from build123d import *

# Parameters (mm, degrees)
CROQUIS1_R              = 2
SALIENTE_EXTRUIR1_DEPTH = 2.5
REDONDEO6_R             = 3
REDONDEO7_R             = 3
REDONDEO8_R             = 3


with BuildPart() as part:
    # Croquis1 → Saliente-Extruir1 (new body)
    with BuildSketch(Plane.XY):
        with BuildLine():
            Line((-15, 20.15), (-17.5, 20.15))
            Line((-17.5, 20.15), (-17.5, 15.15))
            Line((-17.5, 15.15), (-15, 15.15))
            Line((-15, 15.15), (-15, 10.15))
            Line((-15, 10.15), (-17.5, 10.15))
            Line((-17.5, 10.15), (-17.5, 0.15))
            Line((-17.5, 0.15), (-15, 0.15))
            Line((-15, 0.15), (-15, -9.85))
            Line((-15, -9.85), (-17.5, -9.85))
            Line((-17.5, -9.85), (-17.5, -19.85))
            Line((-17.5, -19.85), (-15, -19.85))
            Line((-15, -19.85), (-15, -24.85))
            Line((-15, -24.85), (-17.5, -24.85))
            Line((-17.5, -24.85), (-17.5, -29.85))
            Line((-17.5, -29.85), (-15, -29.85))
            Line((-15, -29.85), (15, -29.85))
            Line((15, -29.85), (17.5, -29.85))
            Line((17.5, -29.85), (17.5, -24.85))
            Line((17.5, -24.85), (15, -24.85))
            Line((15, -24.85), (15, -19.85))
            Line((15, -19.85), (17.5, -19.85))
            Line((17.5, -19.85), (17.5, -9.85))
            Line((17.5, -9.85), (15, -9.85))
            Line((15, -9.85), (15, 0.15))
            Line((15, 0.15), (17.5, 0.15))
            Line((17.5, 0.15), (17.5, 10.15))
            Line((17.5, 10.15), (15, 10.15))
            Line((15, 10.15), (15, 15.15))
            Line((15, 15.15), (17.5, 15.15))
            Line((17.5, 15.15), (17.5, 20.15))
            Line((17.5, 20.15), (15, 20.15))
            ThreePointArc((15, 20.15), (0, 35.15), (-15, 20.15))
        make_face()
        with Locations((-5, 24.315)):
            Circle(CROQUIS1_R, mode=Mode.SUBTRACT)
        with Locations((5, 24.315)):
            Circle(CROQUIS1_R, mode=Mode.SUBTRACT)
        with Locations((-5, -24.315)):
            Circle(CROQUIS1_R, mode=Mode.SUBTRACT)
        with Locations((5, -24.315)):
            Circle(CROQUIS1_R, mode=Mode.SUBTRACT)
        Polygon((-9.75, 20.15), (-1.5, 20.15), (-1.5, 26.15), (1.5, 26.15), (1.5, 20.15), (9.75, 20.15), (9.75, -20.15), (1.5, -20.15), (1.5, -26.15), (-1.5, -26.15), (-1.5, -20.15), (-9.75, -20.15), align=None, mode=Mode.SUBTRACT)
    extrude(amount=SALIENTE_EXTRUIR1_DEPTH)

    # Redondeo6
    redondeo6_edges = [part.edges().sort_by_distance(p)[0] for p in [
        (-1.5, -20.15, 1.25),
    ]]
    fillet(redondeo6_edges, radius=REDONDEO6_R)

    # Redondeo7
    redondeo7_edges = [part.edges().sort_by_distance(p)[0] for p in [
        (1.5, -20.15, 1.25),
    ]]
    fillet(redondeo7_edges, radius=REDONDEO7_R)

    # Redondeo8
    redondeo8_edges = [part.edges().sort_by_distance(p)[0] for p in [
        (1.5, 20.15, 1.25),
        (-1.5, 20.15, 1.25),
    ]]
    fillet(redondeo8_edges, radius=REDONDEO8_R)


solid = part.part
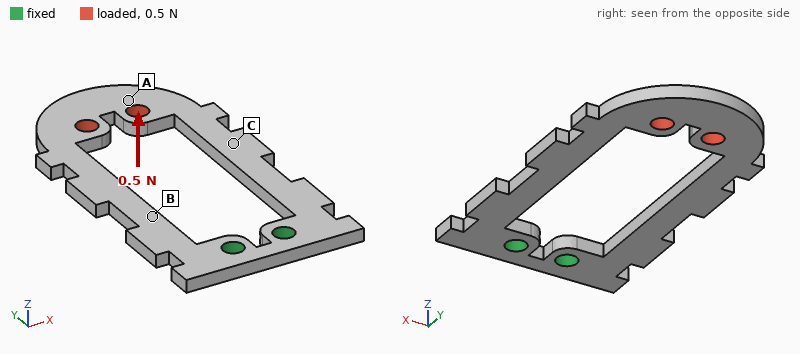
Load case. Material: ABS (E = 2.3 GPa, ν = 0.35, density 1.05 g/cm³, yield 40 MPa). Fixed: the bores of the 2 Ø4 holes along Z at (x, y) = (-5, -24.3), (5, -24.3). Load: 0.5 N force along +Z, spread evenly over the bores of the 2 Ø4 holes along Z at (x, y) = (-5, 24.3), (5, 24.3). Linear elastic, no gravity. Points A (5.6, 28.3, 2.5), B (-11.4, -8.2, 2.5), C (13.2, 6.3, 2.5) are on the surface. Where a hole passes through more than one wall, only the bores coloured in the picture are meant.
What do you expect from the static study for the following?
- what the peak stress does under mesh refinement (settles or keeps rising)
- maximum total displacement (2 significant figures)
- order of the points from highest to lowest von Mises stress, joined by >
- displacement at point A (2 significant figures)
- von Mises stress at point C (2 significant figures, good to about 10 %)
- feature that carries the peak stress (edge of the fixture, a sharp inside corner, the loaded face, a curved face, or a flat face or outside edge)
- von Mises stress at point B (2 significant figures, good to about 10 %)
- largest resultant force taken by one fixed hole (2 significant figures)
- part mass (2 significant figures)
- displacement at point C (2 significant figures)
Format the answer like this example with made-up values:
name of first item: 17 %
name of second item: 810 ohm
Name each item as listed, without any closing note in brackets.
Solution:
what the peak stress does under mesh refinement: keeps rising
maximum total displacement: 0.75 mm
order of the points from highest to lowest von Mises stress, joined by >: B > C > A
displacement at point A: 0.63 mm
von Mises stress at point C: 0.60 MPa
feature that carries the peak stress: a sharp inside corner
von Mises stress at point B: 1.4 MPa
largest resultant force taken by one fixed hole: 0.25 N
part mass: 2.9 g
displacement at point C: 0.27 mm
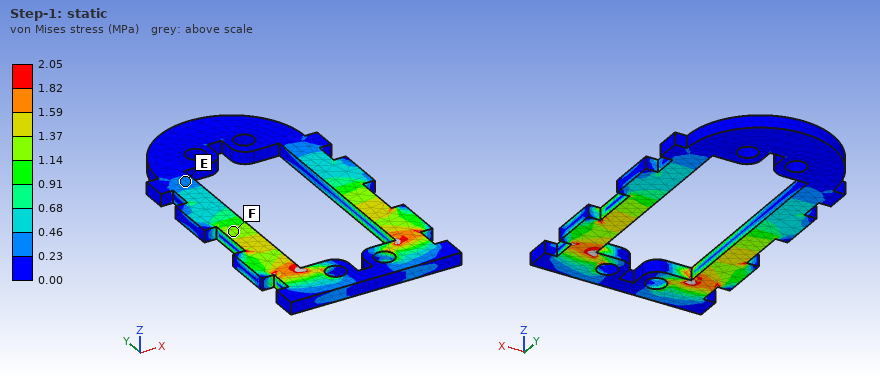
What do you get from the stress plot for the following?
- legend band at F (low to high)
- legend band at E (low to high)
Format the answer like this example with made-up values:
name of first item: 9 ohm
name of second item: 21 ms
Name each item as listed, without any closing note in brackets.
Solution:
legend band at F: 1.14 to 1.37 MPa
legend band at E: 0.23 to 0.46 MPa
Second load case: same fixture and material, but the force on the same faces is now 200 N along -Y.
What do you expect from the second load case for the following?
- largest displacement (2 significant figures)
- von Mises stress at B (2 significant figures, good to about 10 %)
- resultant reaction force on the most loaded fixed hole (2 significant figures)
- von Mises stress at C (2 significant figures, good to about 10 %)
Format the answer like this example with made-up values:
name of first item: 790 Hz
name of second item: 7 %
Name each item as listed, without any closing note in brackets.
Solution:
largest displacement: 0.44 mm
von Mises stress at B: 8.3 MPa
resultant reaction force on the most loaded fixed hole: 110 N
von Mises stress at C: 5.7 MPa
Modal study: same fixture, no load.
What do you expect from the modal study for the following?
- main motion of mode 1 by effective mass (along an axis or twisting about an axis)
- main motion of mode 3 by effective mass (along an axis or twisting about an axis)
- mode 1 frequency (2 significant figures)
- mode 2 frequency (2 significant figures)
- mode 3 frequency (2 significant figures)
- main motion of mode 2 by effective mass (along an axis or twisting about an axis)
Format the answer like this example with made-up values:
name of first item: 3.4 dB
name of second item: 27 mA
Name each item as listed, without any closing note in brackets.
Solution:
main motion of mode 1 by effective mass: along Z
main motion of mode 3 by effective mass: along X
mode 1 frequency: 130 Hz
mode 2 frequency: 450 Hz
mode 3 frequency: 540 Hz
main motion of mode 2 by effective mass: twisting about Y
